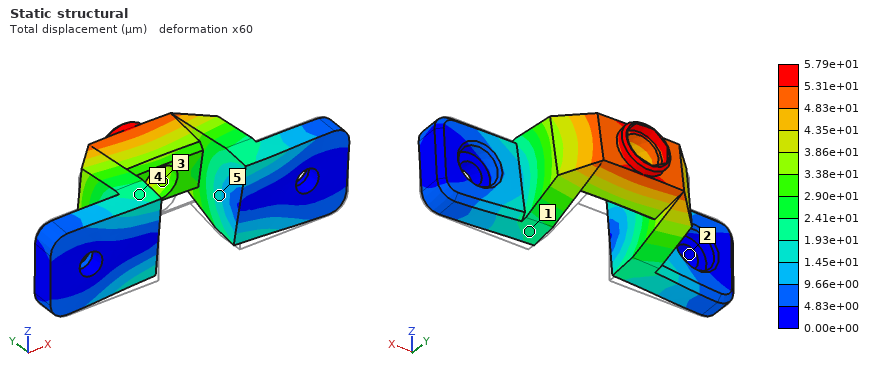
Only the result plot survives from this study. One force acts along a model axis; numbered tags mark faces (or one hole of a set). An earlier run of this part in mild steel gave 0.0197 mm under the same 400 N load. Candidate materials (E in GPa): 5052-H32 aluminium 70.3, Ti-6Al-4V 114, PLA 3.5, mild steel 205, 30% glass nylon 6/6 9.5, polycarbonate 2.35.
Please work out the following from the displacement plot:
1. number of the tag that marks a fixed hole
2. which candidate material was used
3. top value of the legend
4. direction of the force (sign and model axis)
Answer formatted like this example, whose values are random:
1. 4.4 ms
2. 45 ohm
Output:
1. 2
2. 5052-H32 aluminium
3. 5.79e+01 µm
4. +Z
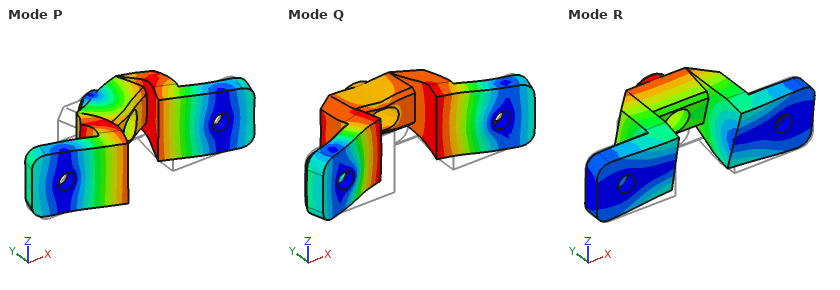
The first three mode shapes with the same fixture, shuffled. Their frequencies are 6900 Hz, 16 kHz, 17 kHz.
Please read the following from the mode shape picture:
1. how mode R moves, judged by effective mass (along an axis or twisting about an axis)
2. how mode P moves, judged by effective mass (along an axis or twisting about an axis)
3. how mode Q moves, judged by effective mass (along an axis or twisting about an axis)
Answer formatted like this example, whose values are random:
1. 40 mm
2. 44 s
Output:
1. along Z
2. along X
3. along Y
